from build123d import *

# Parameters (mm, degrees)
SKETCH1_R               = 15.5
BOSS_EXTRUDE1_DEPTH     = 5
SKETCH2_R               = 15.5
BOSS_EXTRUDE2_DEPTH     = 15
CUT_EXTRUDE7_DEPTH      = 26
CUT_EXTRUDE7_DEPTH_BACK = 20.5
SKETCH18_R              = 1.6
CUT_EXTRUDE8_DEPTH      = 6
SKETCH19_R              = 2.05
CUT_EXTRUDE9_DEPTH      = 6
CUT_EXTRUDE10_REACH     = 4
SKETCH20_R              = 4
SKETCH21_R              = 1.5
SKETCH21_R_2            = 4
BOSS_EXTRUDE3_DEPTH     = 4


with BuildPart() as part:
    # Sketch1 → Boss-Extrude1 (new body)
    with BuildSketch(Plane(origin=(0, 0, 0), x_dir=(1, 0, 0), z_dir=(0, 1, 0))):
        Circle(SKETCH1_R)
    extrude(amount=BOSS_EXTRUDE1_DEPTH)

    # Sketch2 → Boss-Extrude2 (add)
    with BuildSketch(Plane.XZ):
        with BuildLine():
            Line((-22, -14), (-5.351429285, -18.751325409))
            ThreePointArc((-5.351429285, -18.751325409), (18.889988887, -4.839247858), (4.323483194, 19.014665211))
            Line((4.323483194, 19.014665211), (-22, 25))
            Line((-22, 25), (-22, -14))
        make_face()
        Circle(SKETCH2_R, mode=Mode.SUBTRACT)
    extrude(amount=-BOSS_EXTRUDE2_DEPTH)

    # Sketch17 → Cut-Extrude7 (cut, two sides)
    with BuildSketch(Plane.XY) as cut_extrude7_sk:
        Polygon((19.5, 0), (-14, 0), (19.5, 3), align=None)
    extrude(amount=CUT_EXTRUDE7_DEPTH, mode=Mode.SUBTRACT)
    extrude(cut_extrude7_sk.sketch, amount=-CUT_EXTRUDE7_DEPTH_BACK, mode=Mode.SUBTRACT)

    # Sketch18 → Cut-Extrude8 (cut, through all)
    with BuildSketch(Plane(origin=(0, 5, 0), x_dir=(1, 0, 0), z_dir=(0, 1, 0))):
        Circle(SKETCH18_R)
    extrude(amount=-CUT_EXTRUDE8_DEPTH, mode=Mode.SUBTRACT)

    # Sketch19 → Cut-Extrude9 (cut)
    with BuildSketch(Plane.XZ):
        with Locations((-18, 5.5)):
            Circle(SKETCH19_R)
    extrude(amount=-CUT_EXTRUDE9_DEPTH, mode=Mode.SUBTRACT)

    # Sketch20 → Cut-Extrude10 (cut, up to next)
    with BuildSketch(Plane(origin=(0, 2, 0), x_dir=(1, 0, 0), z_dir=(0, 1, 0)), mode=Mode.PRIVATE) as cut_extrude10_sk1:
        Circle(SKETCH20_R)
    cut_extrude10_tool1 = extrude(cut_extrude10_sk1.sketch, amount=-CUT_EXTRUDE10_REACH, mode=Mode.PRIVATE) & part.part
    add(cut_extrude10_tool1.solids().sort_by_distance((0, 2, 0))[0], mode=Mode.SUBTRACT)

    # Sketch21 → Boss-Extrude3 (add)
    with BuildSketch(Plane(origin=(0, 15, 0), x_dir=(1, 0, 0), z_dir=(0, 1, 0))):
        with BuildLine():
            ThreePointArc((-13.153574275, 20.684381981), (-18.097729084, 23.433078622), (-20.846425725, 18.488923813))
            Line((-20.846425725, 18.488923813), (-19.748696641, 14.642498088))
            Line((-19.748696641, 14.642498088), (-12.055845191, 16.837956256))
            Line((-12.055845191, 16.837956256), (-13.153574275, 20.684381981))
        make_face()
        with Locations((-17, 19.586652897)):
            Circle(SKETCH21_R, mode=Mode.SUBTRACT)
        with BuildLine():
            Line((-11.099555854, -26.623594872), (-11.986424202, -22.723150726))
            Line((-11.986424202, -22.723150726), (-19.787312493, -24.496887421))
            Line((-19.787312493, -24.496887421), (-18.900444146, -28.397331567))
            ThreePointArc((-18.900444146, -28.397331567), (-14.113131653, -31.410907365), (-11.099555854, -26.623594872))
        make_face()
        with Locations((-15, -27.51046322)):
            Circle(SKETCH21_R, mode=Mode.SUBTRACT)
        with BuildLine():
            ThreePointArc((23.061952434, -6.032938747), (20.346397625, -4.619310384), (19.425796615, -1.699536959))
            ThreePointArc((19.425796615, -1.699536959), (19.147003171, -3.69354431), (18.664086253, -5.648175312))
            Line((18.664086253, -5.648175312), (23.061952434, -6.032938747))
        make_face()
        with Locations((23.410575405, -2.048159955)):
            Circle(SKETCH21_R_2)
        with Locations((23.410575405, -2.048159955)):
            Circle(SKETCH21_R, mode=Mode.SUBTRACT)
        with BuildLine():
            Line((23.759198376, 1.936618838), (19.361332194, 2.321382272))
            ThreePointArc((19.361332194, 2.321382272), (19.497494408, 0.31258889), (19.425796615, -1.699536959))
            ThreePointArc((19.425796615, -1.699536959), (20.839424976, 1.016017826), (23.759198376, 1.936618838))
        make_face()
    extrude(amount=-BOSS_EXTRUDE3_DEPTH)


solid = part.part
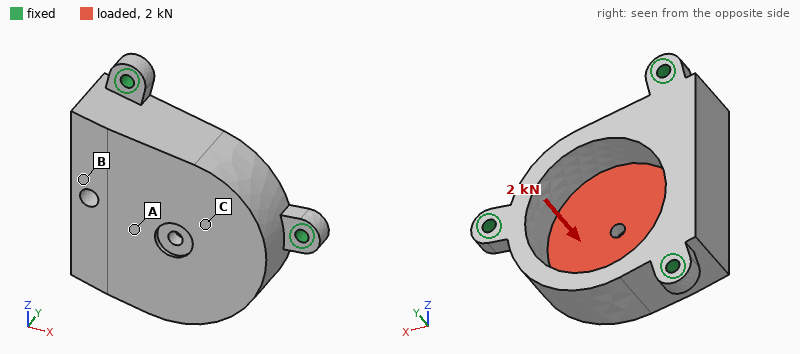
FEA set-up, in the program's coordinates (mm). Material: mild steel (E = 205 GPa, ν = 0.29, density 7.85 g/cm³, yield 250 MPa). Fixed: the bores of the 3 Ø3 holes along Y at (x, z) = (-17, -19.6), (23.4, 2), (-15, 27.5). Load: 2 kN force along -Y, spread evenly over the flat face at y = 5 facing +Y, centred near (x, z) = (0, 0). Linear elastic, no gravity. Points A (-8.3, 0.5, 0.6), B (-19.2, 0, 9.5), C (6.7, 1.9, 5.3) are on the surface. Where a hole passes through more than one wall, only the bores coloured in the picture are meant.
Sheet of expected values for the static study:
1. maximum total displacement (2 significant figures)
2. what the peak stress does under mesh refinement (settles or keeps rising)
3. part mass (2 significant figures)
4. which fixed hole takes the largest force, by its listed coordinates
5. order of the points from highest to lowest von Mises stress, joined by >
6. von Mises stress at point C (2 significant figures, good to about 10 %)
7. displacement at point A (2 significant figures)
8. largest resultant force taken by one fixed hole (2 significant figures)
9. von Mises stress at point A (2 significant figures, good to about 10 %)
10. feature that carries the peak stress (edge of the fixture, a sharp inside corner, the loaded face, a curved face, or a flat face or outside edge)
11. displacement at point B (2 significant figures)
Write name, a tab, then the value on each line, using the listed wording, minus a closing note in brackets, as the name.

maximum total displacement	11 µm
what the peak stress does under mesh refinement	keeps rising
part mass	110 g
which fixed hole takes the largest force, by its listed coordinates	(23.4, 2)
order of the points from highest to lowest von Mises stress, joined by >	C > A > B
von Mises stress at point C	33 MPa
displacement at point A	6.8 µm
largest resultant force taken by one fixed hole	1.0 kN
von Mises stress at point A	24 MPa
feature that carries the peak stress	edge of the fixture
displacement at point B	2.5 µm
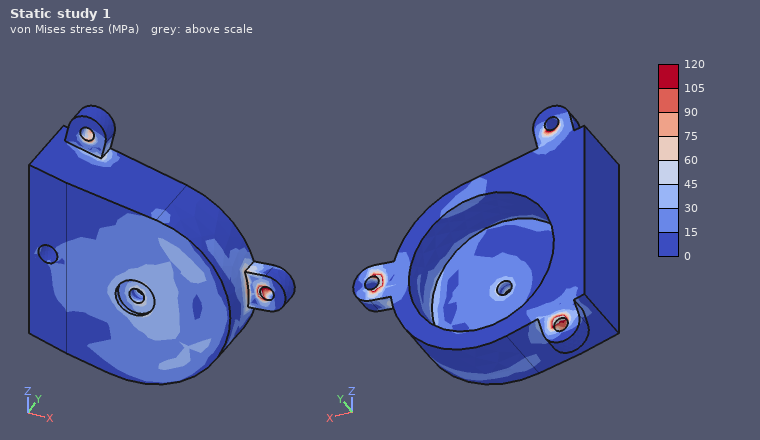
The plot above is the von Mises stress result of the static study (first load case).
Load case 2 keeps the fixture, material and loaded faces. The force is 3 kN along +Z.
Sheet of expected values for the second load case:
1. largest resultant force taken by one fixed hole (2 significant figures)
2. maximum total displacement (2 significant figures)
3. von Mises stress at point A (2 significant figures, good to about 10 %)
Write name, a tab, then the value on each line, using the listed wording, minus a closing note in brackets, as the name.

largest resultant force taken by one fixed hole	1.2 kN
maximum total displacement	6.2 µm
von Mises stress at point A	14 MPa
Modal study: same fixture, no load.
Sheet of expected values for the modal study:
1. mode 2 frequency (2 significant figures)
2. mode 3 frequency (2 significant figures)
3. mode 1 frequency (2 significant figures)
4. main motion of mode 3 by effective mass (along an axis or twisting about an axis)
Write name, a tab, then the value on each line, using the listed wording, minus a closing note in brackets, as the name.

mode 2 frequency	12 kHz
mode 3 frequency	13 kHz
mode 1 frequency	12 kHz
main motion of mode 3 by effective mass	along X
